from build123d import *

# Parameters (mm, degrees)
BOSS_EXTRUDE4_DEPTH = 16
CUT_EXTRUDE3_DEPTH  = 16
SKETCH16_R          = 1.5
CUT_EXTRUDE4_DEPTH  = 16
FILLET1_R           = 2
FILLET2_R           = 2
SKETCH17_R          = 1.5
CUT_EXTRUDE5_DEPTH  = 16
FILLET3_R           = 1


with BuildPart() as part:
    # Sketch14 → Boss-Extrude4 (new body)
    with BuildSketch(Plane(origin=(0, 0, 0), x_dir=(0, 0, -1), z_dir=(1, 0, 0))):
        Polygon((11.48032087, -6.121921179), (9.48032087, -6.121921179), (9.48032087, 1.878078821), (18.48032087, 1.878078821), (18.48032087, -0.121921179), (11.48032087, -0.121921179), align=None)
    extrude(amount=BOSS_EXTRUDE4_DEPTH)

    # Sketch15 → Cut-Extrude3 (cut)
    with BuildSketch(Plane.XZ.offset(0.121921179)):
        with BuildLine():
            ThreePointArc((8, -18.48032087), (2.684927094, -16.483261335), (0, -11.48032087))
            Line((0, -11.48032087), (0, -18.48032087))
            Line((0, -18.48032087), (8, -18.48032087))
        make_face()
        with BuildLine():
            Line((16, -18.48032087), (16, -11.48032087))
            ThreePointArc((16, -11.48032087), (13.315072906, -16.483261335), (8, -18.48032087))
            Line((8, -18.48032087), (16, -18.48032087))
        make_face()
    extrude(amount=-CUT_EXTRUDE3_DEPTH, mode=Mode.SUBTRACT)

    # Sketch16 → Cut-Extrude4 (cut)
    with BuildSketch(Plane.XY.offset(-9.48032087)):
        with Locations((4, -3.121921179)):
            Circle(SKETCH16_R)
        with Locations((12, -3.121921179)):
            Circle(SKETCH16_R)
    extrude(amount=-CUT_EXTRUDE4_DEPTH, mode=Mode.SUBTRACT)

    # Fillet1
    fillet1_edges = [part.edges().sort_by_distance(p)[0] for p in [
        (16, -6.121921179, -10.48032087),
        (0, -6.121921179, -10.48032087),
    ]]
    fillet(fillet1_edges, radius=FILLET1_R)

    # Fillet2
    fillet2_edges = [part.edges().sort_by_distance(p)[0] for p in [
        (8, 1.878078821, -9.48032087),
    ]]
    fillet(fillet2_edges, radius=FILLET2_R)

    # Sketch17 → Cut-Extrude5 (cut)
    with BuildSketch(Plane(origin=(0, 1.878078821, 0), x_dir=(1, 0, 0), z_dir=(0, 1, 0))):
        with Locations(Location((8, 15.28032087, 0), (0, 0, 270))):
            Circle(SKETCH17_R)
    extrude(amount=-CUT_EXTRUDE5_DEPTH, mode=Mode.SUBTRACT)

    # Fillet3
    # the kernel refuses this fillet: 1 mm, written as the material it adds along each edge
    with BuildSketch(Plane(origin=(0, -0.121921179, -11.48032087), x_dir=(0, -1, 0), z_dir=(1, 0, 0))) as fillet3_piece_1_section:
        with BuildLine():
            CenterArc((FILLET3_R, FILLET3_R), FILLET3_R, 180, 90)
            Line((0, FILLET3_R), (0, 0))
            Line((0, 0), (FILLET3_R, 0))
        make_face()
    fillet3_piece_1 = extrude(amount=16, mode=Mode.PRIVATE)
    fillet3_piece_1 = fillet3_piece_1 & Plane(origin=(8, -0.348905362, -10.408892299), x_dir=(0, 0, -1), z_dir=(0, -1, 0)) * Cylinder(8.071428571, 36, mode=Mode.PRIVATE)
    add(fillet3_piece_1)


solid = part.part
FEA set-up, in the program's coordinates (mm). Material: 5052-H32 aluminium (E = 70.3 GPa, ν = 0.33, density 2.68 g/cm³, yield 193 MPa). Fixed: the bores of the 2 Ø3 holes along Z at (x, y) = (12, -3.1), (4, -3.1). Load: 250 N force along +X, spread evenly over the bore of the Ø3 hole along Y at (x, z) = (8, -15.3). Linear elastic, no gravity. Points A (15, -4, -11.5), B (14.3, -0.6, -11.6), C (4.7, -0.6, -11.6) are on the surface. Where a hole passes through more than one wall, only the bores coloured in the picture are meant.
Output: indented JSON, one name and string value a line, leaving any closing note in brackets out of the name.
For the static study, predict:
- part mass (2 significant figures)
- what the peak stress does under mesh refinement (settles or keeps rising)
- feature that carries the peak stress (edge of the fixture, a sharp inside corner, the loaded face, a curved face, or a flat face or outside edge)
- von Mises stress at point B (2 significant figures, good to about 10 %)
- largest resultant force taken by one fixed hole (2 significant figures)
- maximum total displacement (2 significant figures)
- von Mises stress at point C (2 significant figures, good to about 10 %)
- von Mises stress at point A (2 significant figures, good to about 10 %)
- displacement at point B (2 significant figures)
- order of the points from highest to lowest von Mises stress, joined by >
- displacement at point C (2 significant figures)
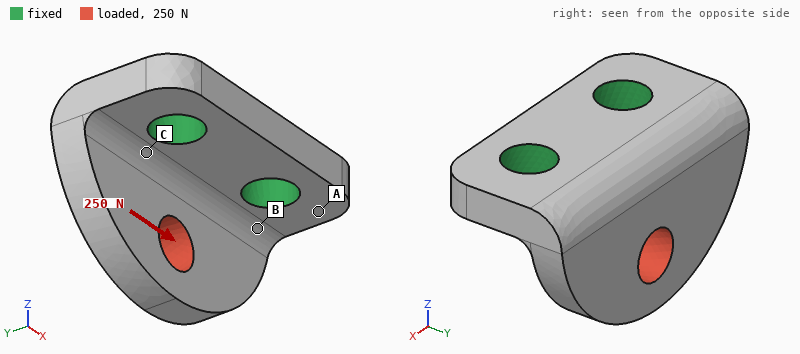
{
  "part mass": "0.99 g",
  "what the peak stress does under mesh refinement": "keeps rising",
  "feature that carries the peak stress": "edge of the fixture",
  "von Mises stress at point B": "31 MPa",
  "largest resultant force taken by one fixed hole": "190 N",
  "maximum total displacement": "9.0 µm",
  "von Mises stress at point C": "54 MPa",
  "von Mises stress at point A": "10 MPa",
  "displacement at point B": "2.9 µm",
  "order of the points from highest to lowest von Mises stress, joined by >": "C > B > A",
  "displacement at point C": "1.5 µm"
}
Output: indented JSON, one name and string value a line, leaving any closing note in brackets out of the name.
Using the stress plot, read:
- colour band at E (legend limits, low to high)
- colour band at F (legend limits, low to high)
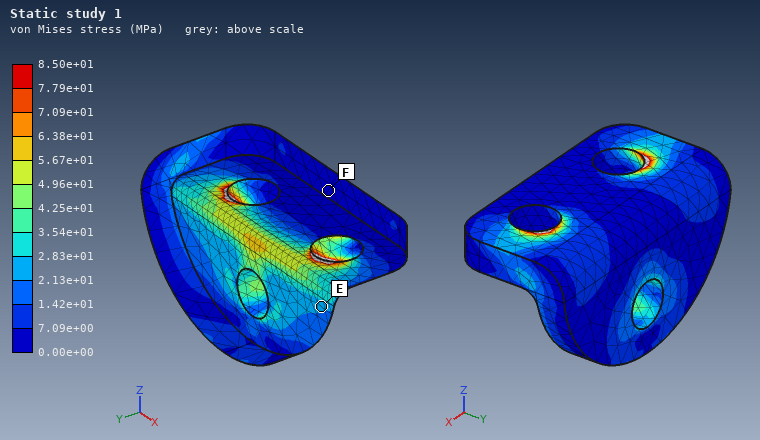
{
  "colour band at E": "2.13e+01 to 2.83e+01 MPa",
  "colour band at F": "0.00e+00 to 7.09e+00 MPa"
}
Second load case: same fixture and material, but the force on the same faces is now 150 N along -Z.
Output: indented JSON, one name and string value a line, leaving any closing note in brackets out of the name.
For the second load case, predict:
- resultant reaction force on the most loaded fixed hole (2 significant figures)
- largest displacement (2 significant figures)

{
  "resultant reaction force on the most loaded fixed hole": "76 N",
  "largest displacement": "9.7 µm"
}
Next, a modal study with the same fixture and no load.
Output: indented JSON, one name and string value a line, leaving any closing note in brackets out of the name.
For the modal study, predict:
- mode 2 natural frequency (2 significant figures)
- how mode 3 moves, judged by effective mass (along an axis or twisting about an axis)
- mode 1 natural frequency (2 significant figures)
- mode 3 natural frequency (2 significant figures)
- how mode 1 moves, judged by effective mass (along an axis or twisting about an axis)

{
  "mode 2 natural frequency": "40 kHz",
  "how mode 3 moves, judged by effective mass": "along X",
  "mode 1 natural frequency": "24 kHz",
  "mode 3 natural frequency": "63 kHz",
  "how mode 1 moves, judged by effective mass": "along Y"
}
